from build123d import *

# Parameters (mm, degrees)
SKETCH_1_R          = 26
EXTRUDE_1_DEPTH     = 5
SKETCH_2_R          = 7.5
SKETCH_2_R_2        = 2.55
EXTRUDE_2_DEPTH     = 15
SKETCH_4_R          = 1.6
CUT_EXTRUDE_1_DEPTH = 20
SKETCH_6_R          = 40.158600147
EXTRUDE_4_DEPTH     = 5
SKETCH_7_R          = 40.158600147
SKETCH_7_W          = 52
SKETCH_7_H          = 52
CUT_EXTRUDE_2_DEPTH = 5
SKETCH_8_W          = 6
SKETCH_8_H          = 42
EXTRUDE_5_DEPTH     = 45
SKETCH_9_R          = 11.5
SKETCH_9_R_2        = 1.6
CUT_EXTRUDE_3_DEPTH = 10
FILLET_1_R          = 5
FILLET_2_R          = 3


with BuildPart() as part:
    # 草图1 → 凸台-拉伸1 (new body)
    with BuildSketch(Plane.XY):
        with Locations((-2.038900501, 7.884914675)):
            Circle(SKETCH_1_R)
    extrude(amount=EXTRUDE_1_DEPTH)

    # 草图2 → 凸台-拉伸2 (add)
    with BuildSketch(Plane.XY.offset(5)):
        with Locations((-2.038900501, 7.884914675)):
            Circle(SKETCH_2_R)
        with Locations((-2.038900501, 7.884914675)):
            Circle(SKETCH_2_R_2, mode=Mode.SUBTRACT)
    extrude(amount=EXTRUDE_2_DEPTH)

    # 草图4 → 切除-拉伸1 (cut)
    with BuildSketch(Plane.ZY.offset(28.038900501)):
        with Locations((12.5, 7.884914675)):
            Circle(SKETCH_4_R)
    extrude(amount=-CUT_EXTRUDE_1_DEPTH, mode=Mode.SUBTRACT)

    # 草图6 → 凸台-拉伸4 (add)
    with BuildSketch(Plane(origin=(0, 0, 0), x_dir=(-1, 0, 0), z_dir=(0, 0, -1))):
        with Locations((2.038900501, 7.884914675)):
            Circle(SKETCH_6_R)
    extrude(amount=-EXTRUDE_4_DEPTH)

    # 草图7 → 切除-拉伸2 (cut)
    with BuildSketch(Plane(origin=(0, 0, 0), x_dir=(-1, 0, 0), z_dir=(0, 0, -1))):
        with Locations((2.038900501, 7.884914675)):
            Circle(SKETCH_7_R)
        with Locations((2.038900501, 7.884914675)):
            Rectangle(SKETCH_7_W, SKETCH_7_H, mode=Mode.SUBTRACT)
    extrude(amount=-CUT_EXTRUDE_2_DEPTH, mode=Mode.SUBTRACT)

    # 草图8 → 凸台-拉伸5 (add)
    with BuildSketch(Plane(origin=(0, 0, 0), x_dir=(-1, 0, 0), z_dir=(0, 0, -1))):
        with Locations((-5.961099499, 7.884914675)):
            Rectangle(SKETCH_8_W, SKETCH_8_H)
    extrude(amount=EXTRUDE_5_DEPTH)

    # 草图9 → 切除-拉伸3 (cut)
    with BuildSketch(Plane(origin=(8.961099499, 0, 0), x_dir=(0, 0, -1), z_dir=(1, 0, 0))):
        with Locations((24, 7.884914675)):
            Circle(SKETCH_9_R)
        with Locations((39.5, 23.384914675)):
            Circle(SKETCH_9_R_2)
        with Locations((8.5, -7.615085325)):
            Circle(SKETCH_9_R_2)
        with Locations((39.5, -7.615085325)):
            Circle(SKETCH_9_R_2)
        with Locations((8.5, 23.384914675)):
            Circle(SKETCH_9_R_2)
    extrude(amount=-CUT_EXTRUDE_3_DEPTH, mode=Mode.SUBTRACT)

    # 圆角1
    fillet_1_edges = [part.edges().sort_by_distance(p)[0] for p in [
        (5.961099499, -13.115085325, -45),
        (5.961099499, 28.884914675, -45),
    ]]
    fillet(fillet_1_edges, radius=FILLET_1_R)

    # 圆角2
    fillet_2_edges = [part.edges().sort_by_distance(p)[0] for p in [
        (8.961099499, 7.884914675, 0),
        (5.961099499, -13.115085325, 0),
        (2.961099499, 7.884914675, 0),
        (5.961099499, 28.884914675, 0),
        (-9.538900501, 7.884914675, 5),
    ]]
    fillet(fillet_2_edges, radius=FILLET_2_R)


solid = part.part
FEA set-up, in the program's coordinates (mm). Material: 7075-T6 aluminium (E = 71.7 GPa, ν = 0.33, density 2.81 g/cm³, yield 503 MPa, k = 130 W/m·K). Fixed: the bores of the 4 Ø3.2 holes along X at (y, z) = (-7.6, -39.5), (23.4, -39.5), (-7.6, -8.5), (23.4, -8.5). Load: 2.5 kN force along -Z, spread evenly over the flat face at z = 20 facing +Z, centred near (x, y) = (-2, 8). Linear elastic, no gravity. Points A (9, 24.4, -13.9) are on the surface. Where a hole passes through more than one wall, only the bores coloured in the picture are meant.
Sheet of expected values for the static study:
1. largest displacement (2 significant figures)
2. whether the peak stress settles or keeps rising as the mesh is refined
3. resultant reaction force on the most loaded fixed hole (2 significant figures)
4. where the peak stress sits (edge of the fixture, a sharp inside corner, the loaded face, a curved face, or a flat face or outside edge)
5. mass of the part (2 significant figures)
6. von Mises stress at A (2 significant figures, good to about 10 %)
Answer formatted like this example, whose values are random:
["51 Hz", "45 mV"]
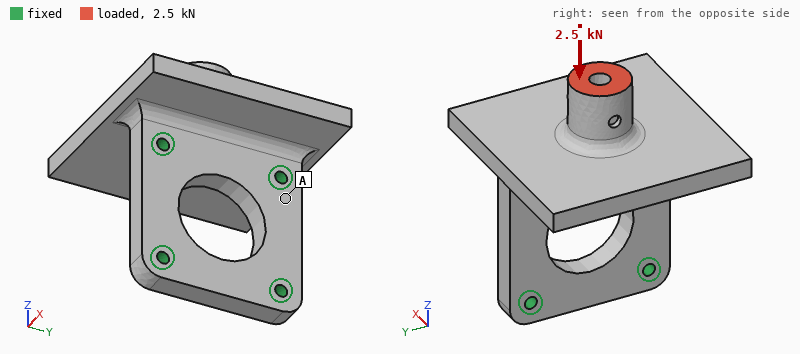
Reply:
["0.17 mm", "keeps rising", "1.3 kN", "edge of the fixture", "70 g", "19 MPa"]
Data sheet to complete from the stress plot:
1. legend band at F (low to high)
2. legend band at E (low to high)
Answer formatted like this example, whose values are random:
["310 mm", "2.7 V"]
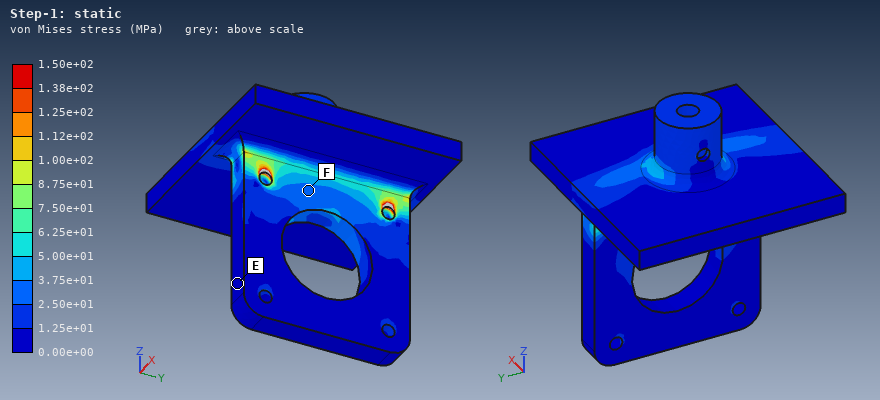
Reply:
["2.50e+01 to 3.75e+01 MPa", "0.00e+00 to 1.25e+01 MPa"]
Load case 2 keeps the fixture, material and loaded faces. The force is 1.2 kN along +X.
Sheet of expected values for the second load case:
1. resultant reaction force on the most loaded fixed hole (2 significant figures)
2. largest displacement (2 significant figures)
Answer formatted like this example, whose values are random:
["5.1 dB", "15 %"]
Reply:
["710 N", "0.26 mm"]
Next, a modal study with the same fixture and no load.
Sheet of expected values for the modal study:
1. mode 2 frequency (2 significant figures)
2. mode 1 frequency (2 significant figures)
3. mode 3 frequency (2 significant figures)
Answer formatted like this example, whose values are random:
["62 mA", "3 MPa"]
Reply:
["5600 Hz", "2600 Hz", "7600 Hz"]
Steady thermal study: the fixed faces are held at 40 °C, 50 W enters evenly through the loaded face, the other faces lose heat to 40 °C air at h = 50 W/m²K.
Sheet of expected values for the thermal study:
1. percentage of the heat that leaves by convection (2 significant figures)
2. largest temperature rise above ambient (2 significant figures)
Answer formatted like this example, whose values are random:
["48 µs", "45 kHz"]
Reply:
["17 %", "64 K"]
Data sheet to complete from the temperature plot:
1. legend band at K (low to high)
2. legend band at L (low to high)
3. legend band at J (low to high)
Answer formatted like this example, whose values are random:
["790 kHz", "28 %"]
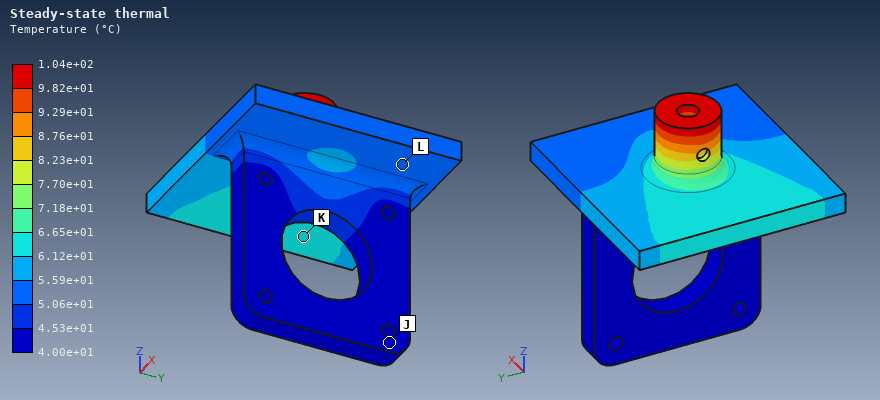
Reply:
["6.12e+01 to 6.65e+01 °C", "5.06e+01 to 5.59e+01 °C", "4.00e+01 to 4.53e+01 °C"]
